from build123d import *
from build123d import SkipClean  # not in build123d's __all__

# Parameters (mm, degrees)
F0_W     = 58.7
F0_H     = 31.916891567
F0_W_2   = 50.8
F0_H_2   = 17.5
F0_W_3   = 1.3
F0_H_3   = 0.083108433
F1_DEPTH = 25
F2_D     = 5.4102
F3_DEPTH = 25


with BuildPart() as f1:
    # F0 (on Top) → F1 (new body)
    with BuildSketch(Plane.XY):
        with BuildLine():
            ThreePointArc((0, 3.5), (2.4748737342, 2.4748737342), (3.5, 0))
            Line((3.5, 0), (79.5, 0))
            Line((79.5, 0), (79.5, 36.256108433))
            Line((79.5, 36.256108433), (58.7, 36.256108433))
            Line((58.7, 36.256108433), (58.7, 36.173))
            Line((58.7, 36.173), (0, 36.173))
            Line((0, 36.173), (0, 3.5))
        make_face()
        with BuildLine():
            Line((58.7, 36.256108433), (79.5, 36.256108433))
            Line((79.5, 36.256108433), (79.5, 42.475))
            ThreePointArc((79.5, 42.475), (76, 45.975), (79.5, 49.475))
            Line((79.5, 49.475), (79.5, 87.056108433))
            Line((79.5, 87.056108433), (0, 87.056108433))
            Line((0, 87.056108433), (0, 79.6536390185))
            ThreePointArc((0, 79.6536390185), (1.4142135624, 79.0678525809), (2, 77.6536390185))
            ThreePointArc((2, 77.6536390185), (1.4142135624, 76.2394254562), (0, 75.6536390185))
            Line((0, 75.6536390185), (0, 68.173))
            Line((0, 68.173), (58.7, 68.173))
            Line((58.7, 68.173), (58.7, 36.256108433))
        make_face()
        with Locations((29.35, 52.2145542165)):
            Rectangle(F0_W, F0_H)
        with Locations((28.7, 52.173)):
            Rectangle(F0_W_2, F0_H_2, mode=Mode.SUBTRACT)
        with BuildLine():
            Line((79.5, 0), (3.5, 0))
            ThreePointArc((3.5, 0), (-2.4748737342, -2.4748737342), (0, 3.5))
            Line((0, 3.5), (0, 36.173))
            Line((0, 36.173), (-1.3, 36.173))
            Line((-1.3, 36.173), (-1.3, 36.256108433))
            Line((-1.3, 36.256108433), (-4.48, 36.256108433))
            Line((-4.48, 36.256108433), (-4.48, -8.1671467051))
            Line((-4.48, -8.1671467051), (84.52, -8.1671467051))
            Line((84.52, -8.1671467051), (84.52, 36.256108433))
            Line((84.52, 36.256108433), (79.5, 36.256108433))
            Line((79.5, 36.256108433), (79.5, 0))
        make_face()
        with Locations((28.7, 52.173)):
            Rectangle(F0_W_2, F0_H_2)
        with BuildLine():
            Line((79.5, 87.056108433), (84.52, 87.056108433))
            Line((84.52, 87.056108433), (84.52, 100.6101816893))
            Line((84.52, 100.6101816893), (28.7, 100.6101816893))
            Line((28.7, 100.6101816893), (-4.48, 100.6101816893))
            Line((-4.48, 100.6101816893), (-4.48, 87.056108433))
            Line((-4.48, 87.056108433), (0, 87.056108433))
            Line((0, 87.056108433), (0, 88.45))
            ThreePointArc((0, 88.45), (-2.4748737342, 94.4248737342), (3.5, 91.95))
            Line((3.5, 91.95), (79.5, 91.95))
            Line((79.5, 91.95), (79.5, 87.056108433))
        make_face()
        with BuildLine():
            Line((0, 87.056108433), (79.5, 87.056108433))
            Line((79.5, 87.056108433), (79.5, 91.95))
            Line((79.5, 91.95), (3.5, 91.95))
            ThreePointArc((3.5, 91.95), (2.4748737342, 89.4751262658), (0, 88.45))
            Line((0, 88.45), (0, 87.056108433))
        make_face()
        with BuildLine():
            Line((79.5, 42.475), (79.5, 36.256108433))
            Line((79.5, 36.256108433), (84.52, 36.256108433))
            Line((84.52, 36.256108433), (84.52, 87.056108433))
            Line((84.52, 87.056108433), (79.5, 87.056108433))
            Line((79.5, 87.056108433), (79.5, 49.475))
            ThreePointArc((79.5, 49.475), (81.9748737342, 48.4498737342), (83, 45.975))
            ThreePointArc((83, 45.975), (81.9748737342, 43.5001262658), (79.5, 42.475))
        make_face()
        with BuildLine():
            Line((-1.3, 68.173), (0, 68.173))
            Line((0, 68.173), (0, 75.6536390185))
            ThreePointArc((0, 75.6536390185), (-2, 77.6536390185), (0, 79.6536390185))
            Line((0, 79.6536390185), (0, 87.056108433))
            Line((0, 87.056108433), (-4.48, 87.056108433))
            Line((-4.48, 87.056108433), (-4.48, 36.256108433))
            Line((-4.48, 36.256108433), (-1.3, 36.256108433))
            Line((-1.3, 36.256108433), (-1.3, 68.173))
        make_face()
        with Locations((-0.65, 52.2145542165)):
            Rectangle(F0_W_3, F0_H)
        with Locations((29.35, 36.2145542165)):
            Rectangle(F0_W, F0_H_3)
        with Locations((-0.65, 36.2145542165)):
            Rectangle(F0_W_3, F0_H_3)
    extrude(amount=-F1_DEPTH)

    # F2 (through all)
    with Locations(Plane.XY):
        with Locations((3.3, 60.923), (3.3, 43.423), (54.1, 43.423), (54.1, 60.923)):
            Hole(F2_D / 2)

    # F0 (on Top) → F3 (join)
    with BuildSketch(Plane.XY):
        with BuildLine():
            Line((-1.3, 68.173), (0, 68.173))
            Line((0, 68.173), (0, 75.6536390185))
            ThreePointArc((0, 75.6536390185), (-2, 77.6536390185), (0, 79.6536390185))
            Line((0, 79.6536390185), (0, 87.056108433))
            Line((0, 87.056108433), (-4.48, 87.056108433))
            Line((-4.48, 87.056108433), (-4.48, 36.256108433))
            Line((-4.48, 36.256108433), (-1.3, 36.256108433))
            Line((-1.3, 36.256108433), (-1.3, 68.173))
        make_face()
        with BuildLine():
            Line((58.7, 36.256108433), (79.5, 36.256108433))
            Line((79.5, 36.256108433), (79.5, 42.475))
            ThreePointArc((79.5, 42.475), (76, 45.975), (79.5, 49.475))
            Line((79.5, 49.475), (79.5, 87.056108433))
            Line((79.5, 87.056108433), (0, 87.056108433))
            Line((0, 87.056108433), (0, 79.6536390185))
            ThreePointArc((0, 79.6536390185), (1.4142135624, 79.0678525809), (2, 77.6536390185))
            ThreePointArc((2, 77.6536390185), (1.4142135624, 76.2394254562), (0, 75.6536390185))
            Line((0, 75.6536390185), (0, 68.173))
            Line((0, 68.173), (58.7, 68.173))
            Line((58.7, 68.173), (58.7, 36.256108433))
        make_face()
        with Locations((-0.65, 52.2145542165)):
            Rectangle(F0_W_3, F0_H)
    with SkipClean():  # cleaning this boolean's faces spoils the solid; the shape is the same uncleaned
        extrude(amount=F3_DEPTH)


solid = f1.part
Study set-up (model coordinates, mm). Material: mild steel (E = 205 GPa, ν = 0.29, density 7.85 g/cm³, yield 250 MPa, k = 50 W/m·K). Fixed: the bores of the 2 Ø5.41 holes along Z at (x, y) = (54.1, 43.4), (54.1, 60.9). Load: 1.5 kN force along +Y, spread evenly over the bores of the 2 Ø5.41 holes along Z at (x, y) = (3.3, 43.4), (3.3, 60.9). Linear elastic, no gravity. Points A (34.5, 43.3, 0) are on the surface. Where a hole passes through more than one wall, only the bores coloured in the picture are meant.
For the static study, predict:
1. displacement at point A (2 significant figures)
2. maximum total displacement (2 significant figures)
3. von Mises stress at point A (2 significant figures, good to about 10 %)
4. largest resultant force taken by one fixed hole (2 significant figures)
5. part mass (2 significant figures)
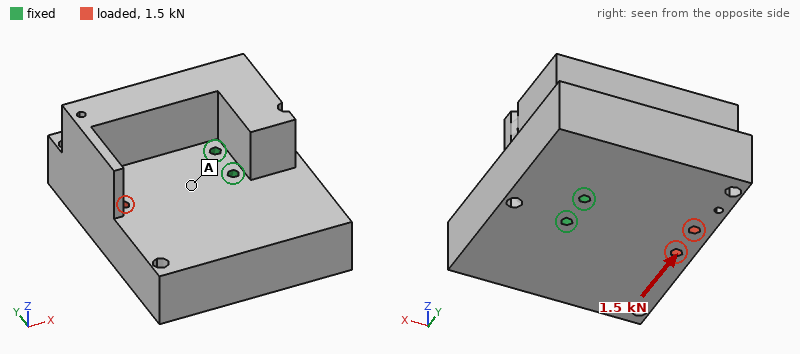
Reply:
1.1 µm
4.3 µm
3.0 MPa
3.6 kN
2.3 kg
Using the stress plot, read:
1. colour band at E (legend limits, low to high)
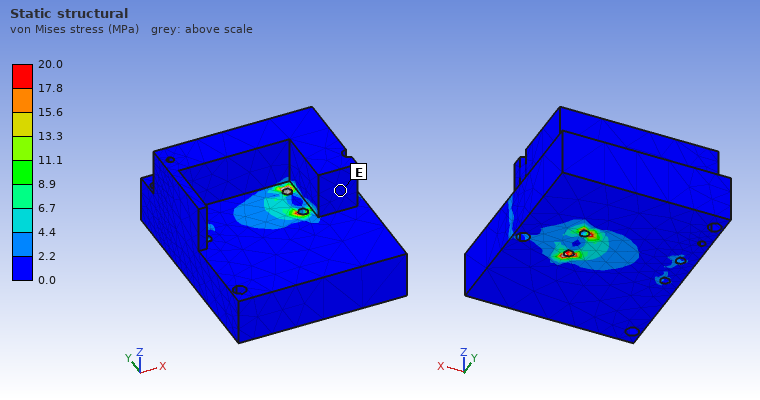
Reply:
0.0 to 2.2 MPa
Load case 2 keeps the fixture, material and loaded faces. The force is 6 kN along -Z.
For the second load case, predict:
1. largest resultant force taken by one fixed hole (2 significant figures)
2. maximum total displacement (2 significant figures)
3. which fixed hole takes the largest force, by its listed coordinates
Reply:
3.3 kN
24 µm
(54.1, 60.9)
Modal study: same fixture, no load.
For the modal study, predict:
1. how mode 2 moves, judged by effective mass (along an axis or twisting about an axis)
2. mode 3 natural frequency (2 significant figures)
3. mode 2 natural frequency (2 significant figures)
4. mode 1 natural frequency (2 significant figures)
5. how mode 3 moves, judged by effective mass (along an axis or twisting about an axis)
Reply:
along Z
4000 Hz
3500 Hz
3200 Hz
twisting about X
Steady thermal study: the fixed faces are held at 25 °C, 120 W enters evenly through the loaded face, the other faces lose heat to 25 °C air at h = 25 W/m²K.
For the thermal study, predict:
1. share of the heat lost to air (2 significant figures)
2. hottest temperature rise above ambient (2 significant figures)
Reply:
20 %
70 K
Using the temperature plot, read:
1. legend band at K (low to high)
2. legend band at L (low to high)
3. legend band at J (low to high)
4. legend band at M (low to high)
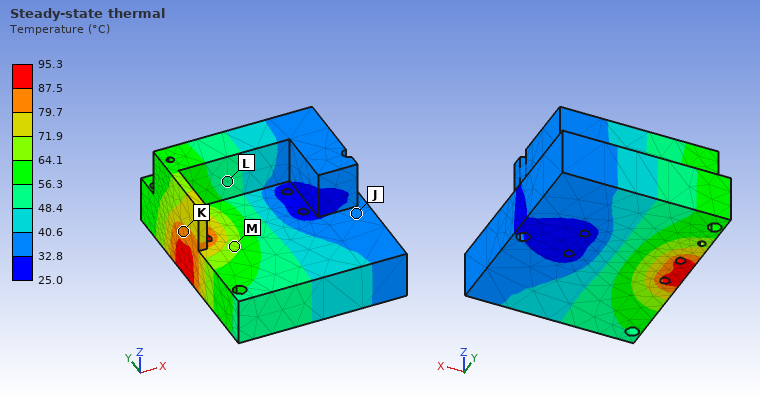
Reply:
79.7 to 87.5 °C
48.4 to 56.3 °C
32.8 to 40.6 °C
64.1 to 71.9 °C
